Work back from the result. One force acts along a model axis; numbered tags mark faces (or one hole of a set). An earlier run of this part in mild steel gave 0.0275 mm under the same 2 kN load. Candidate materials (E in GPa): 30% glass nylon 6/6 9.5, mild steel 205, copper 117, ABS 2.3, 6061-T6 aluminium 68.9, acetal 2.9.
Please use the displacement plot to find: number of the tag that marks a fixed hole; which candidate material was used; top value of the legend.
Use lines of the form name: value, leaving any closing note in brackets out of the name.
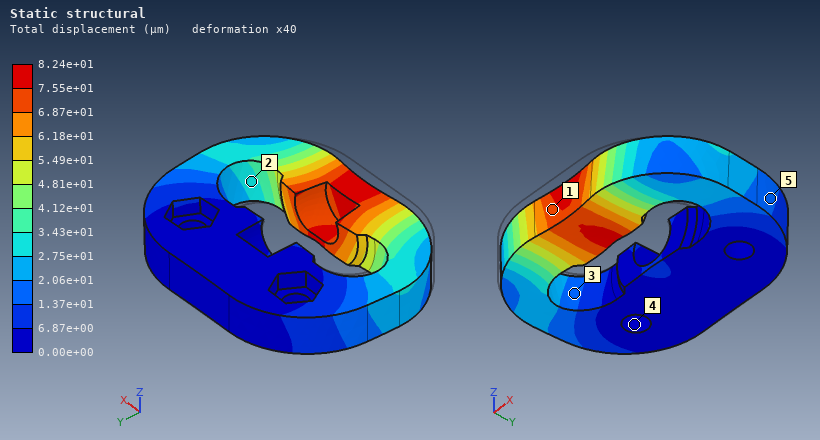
number of the tag that marks a fixed hole: 4
which candidate material was used: 6061-T6 aluminium
top value of the legend: 8.24e+01 µm
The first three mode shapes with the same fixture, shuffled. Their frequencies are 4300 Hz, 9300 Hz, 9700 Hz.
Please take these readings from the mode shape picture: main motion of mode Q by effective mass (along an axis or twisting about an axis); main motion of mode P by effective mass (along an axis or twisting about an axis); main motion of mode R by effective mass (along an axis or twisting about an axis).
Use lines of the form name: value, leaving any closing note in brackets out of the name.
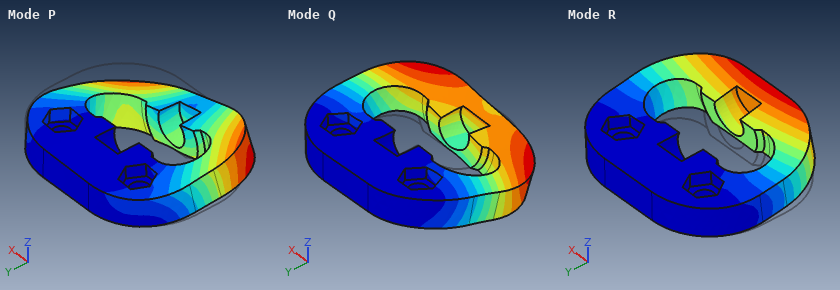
main motion of mode Q by effective mass: along X
main motion of mode P by effective mass: along X
main motion of mode R by effective mass: along Z
